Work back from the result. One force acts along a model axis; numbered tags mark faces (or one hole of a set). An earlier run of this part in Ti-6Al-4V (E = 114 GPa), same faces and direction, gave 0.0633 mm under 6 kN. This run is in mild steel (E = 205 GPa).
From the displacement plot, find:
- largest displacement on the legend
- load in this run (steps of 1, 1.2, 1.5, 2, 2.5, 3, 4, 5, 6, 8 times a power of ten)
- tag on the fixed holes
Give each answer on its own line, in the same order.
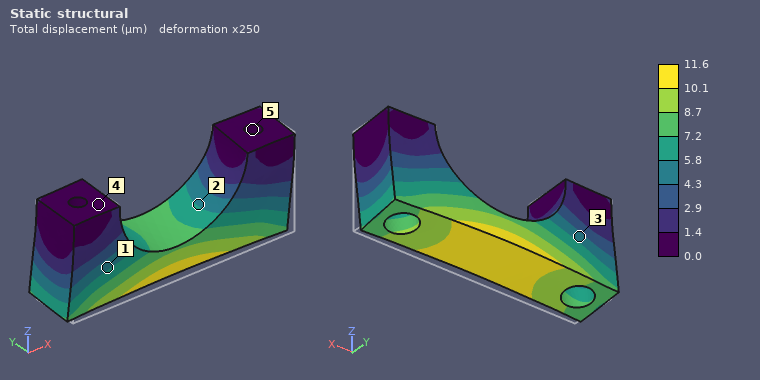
11.6 µm
2 kN
5
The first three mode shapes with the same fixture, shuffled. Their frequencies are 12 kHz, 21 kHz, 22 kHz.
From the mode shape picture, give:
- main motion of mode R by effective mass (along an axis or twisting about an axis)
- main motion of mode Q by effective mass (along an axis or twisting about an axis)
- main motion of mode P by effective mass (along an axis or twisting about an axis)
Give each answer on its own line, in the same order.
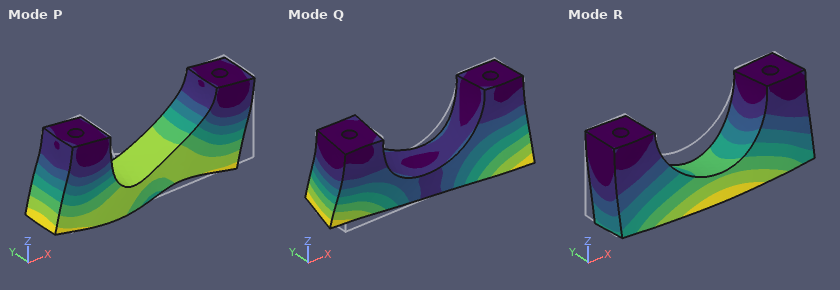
along Y
twisting about Z
along X
